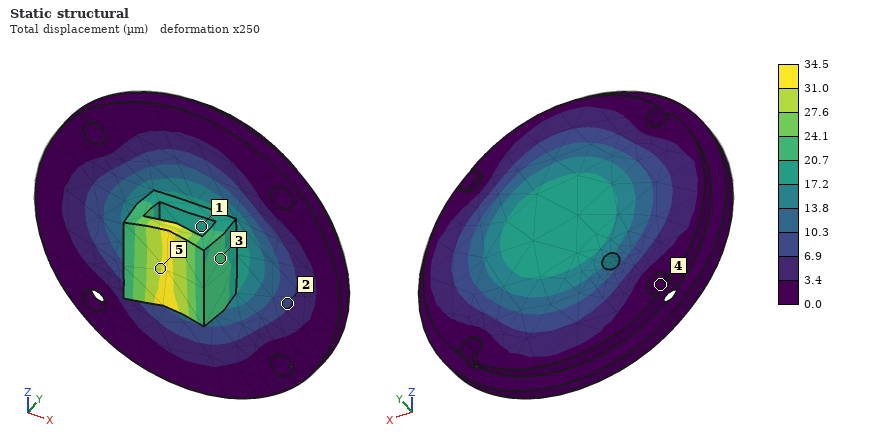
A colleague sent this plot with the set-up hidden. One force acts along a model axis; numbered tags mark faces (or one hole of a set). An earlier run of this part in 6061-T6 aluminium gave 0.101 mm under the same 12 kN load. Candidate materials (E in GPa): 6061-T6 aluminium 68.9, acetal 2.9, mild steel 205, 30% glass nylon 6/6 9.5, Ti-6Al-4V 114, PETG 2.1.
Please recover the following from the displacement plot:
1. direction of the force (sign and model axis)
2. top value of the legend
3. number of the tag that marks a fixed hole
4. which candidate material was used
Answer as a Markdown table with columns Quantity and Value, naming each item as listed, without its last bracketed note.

| Quantity | Value |
|---|---|
| direction of the force | +Y |
| top value of the legend | 34.5 µm |
| number of the tag that marks a fixed hole | 4 |
| which candidate material was used | mild steel |
